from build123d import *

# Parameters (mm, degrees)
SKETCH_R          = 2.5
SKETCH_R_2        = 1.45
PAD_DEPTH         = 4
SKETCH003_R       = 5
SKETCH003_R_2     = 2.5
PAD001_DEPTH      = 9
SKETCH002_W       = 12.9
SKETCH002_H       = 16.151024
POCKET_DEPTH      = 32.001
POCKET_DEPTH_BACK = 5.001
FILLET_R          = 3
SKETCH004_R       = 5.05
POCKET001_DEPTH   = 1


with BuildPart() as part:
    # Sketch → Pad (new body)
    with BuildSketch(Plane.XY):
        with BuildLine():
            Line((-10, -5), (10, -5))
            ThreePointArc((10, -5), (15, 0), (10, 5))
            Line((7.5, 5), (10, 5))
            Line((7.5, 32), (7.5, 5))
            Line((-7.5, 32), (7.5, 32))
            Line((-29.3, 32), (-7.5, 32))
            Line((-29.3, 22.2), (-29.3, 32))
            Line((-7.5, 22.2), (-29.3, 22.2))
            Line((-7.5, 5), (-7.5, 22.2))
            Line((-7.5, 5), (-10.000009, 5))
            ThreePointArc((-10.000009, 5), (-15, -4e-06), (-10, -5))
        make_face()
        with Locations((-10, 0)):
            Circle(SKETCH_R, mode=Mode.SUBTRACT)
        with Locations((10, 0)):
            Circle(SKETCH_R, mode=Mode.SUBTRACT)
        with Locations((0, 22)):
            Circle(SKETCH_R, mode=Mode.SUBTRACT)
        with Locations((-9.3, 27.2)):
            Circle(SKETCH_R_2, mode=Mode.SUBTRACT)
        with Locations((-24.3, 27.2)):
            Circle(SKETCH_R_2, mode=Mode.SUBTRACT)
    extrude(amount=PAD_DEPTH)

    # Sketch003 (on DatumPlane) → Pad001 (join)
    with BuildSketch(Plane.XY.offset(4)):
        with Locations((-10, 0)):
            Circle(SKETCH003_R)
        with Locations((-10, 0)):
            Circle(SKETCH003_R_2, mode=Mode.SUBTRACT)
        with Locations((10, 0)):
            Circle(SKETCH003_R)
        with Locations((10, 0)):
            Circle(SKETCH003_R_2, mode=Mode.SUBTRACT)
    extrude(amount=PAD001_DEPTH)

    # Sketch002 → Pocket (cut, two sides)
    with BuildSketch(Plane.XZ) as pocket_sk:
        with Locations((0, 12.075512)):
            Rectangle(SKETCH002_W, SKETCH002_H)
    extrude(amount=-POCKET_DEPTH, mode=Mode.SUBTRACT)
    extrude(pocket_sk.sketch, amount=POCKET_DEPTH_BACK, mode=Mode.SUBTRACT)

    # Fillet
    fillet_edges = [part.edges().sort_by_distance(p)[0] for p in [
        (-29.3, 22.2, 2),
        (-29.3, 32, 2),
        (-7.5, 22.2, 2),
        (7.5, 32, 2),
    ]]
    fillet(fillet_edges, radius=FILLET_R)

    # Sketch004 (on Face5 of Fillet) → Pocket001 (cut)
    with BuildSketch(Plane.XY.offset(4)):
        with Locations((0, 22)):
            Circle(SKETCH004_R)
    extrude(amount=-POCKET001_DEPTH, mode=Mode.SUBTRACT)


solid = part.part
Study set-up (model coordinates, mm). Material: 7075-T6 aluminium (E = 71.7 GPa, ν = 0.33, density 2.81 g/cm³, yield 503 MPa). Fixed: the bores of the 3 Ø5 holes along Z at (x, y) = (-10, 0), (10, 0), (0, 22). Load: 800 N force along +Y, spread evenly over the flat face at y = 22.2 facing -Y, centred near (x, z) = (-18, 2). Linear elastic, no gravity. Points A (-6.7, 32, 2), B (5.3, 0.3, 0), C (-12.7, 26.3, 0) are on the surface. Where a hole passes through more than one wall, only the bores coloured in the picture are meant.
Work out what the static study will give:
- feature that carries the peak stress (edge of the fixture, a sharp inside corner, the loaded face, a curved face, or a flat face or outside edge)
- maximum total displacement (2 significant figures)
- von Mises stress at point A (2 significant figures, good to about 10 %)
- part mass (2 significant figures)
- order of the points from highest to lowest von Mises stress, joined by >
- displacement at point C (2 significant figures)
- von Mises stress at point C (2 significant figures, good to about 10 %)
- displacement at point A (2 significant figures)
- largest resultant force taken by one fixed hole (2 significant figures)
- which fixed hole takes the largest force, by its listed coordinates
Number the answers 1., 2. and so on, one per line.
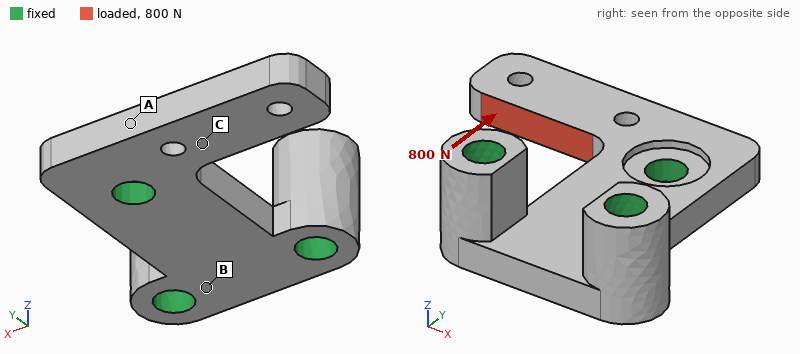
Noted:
1. a curved face
2. 0.13 mm
3. 120 MPa
4. 12 g
5. A > C > B
6. 0.038 mm
7. 53 MPa
8. 0.027 mm
9. 700 N
10. (0, 22)
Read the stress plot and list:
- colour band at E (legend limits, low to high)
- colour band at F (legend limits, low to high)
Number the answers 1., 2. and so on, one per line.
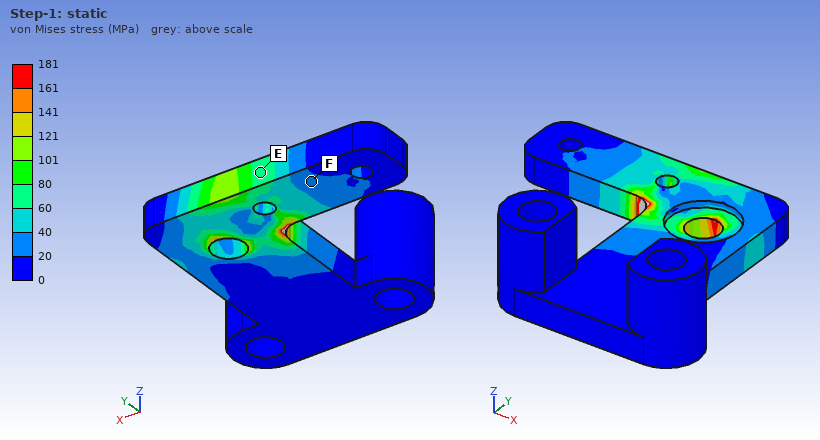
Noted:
1. 60 to 80 MPa
2. 20 to 40 MPa
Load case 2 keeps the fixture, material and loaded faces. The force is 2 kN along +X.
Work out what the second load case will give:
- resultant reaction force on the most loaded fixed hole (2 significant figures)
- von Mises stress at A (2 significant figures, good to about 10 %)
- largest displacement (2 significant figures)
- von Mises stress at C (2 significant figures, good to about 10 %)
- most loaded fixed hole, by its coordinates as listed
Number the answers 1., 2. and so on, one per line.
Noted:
1. 1.9 kN
2. 49 MPa
3. 99 µm
4. 42 MPa
5. (0, 22)
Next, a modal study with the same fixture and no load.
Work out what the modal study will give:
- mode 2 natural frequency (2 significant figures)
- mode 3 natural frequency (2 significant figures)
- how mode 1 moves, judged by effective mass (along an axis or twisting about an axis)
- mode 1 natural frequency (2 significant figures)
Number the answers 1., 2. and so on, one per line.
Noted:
1. 10 kHz
2. 16 kHz
3. along Z
4. 3900 Hz
